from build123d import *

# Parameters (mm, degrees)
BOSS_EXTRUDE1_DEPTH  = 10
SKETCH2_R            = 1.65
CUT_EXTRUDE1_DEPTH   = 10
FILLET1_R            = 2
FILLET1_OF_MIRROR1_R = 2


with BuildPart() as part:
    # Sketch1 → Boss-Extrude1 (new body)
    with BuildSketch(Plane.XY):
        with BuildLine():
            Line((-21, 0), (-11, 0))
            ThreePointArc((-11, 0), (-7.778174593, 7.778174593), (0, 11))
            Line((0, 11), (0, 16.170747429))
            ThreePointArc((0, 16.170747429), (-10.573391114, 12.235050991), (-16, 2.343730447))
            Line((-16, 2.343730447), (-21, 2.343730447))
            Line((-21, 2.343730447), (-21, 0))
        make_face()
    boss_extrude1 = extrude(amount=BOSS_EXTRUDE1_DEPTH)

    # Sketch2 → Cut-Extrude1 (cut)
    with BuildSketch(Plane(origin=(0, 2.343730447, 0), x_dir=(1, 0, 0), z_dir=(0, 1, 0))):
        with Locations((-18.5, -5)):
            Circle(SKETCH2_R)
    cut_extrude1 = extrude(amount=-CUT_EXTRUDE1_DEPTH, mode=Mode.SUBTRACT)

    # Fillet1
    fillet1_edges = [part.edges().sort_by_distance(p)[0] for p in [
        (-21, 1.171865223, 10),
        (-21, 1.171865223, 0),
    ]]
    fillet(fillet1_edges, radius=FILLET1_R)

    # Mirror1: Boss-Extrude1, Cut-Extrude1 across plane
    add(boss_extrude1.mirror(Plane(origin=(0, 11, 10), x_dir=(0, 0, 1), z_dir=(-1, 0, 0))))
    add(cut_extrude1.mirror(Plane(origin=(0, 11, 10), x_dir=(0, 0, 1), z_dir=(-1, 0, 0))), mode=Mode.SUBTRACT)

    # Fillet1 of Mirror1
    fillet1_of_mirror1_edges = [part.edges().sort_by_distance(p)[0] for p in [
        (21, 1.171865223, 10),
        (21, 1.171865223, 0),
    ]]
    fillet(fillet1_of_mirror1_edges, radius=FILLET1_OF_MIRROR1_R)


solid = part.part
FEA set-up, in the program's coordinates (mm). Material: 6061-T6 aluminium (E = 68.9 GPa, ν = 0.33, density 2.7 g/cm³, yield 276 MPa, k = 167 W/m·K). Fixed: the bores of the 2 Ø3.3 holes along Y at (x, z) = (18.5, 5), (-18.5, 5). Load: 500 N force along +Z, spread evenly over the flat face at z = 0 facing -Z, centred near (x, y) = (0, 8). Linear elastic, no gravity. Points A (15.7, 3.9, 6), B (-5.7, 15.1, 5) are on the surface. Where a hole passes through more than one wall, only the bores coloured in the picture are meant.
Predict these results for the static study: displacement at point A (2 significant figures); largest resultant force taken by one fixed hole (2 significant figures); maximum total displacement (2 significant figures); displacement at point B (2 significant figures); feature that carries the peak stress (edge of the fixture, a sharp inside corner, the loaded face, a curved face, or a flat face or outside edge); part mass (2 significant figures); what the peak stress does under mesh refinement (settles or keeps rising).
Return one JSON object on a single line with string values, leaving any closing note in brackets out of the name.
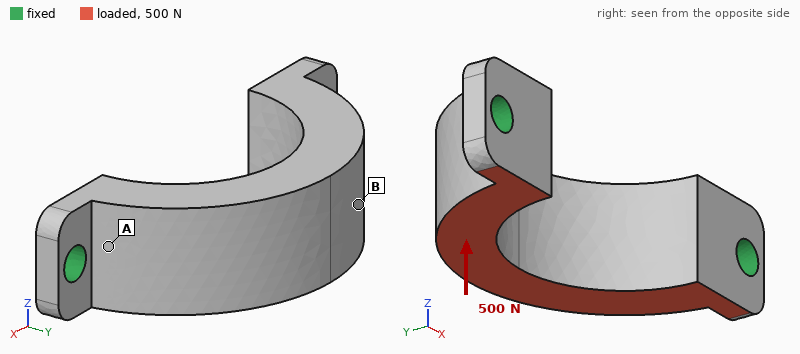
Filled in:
{"displacement at point A": "12 µm", "largest resultant force taken by one fixed hole": "250 N", "maximum total displacement": "65 µm", "displacement at point B": "57 µm", "feature that carries the peak stress": "edge of the fixture", "part mass": "6.4 g", "what the peak stress does under mesh refinement": "keeps rising"}
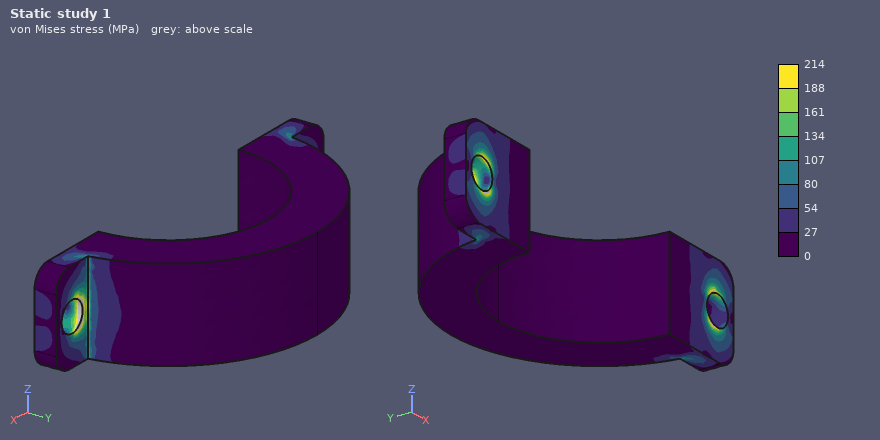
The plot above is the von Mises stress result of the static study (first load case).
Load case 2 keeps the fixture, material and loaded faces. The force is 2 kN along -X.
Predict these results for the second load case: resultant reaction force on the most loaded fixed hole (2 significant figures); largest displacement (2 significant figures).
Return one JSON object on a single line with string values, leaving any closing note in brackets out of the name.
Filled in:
{"resultant reaction force on the most loaded fixed hole": "1.1 kN", "largest displacement": "39 µm"}
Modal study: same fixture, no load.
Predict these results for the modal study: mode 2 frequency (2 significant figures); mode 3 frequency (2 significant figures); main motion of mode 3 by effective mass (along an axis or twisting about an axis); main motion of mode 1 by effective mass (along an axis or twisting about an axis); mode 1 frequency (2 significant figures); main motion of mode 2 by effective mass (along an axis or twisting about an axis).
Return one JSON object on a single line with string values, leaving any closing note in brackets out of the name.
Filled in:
{"mode 2 frequency": "19 kHz", "mode 3 frequency": "25 kHz", "main motion of mode 3 by effective mass": "twisting about Y", "main motion of mode 1 by effective mass": "along Z", "mode 1 frequency": "6700 Hz", "main motion of mode 2 by effective mass": "along X"}
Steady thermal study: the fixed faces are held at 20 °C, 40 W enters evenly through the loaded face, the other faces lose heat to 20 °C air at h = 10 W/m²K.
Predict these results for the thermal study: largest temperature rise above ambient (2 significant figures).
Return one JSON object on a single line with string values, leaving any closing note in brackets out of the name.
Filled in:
{"largest temperature rise above ambient": "40 K"}
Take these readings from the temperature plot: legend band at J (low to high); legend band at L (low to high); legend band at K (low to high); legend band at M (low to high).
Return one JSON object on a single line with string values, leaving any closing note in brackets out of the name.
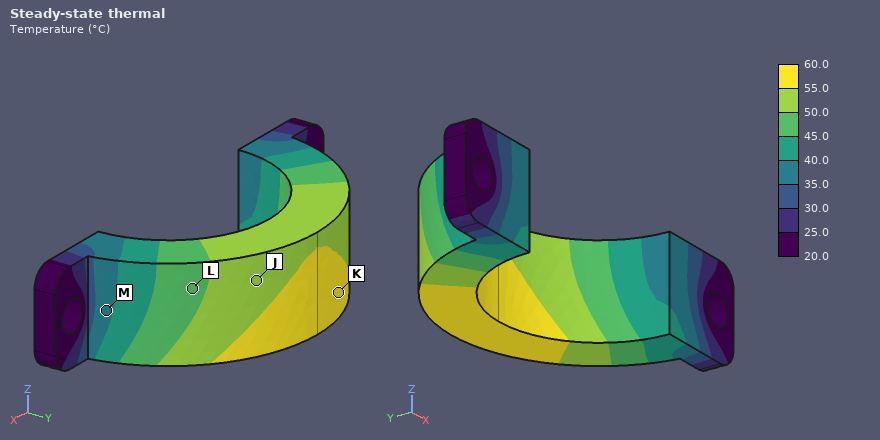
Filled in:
{"legend band at J": "50.0 to 55.0 °C", "legend band at L": "45.0 to 50.0 °C", "legend band at K": "55.0 to 60.0 °C", "legend band at M": "35.0 to 40.0 °C"}
